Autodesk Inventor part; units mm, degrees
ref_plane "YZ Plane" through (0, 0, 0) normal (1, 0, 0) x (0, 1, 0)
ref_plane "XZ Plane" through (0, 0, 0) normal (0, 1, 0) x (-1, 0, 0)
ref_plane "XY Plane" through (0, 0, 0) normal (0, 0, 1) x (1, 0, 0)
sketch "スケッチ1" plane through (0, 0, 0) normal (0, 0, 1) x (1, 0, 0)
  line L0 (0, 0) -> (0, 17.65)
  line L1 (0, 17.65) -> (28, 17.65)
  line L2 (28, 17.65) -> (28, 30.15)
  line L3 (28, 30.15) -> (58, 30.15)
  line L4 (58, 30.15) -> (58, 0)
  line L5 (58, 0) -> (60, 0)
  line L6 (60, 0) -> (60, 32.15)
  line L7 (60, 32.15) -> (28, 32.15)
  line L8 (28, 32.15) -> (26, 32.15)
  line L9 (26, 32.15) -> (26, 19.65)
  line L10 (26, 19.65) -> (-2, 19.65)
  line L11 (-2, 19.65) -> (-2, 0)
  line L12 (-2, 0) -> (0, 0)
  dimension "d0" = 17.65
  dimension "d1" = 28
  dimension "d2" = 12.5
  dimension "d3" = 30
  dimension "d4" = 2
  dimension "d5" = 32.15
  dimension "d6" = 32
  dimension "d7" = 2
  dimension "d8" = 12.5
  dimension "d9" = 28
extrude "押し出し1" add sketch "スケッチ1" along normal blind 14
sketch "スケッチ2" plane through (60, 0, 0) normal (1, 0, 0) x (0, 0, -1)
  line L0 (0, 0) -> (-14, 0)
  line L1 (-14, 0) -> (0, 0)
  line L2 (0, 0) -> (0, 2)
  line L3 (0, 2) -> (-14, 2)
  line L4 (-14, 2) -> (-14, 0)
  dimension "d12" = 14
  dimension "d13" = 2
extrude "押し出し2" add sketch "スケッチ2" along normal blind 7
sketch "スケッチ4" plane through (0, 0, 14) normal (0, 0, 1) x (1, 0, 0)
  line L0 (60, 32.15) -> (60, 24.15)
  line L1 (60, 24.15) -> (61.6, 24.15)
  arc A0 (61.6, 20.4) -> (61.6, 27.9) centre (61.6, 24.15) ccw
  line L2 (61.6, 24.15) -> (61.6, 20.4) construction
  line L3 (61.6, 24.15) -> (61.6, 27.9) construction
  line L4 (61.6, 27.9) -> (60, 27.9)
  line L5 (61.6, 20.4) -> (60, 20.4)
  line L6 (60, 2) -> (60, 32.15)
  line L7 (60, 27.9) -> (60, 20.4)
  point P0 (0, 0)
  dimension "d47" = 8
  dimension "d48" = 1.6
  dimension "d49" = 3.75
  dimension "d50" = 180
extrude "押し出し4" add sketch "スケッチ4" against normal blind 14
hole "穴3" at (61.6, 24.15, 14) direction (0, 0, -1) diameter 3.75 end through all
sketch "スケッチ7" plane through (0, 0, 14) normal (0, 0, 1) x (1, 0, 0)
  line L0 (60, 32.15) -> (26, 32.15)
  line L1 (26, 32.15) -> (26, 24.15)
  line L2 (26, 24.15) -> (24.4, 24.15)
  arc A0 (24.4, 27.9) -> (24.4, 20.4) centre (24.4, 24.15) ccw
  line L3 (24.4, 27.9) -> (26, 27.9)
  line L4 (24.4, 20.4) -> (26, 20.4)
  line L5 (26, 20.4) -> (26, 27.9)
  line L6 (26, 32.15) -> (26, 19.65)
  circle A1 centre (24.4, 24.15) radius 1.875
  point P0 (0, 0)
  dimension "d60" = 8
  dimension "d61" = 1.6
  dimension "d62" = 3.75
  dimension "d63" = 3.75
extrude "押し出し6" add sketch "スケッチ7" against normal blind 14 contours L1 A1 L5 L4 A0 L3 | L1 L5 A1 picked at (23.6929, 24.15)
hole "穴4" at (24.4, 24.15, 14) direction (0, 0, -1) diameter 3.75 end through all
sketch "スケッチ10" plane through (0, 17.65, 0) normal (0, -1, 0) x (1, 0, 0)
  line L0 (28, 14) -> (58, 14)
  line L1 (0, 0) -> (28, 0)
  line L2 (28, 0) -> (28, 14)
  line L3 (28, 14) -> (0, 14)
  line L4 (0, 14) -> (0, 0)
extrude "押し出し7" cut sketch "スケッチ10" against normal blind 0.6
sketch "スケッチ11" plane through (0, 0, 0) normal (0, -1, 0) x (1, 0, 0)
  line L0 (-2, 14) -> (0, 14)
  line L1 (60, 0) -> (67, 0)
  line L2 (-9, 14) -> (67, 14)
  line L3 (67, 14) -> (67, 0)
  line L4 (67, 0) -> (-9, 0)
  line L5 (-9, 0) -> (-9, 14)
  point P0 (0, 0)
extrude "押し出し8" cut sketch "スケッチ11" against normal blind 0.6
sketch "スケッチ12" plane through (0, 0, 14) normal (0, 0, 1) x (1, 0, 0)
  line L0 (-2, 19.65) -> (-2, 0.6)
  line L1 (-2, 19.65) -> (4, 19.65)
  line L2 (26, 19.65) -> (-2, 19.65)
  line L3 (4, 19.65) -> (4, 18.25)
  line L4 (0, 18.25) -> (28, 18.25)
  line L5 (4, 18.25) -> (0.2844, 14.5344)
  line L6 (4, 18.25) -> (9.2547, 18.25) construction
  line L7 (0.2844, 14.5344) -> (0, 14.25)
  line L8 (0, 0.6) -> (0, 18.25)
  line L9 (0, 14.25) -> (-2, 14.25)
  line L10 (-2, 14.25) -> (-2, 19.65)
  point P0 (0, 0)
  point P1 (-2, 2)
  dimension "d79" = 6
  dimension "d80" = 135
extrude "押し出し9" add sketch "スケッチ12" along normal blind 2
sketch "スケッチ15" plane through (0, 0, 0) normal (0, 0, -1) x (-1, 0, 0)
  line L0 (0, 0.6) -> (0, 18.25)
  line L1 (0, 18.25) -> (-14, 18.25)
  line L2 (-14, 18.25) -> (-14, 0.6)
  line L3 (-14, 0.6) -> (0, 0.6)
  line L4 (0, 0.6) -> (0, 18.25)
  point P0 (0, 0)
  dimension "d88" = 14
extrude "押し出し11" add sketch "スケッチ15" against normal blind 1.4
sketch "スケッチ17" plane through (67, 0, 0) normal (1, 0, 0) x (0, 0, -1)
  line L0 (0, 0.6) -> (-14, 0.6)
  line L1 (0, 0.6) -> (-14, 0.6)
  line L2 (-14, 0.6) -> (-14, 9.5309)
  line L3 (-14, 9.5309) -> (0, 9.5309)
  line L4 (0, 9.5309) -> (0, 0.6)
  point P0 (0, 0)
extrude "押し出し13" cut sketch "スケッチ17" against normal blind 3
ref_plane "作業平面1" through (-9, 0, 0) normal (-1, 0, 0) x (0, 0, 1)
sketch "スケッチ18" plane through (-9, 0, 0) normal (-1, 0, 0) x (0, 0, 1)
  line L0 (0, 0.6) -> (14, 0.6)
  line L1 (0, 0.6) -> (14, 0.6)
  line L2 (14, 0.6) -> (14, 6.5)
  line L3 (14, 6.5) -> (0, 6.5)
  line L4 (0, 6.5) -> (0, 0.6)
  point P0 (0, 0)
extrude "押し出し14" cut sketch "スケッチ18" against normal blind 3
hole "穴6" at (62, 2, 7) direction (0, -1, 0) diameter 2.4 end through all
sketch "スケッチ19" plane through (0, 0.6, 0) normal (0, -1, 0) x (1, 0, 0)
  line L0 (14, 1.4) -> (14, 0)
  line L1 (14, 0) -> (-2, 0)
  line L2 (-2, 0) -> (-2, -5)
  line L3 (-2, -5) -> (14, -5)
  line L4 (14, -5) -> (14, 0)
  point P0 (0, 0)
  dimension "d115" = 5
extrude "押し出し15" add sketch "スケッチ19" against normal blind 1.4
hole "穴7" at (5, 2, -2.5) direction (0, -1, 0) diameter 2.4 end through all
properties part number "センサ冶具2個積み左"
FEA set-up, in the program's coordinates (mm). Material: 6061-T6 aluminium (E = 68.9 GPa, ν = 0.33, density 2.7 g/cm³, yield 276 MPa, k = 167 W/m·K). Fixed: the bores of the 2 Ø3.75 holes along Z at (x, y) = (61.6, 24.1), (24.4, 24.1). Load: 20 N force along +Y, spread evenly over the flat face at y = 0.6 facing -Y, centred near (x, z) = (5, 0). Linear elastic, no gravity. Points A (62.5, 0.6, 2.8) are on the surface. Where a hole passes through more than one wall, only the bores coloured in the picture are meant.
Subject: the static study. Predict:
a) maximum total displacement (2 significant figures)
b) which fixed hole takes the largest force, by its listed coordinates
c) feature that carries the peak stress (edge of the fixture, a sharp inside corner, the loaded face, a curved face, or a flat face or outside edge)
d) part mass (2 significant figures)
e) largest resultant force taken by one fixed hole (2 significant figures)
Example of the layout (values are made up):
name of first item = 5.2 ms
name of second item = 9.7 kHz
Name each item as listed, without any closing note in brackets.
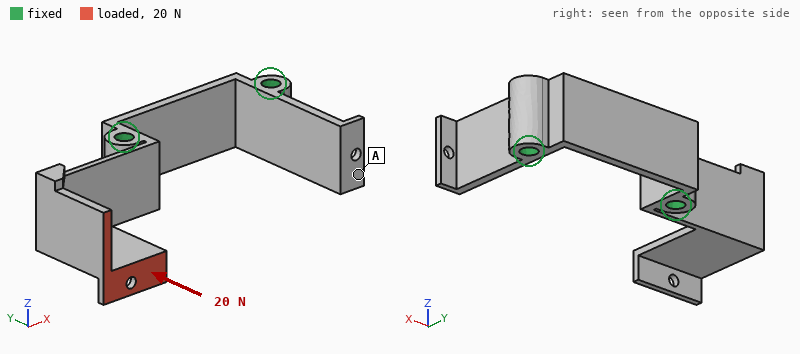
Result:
maximum total displacement = 0.70 mm
which fixed hole takes the largest force, by its listed coordinates = (24.4, 24.1)
feature that carries the peak stress = a flat face or outside edge
part mass = 12 g
largest resultant force taken by one fixed hole = 20 N
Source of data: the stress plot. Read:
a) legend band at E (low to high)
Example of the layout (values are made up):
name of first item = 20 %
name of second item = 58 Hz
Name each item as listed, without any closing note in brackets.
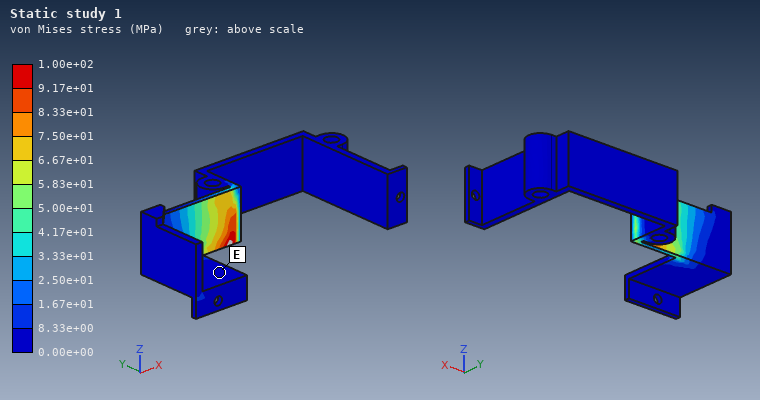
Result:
legend band at E = 0.00e+00 to 8.33e+00 MPa
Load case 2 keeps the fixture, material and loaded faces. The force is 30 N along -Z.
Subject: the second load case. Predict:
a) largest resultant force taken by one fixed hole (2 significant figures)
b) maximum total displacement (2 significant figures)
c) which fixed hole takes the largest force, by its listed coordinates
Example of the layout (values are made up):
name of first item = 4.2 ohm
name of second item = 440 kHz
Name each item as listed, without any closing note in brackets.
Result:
largest resultant force taken by one fixed hole = 30 N
maximum total displacement = 0.62 mm
which fixed hole takes the largest force, by its listed coordinates = (24.4, 24.1)
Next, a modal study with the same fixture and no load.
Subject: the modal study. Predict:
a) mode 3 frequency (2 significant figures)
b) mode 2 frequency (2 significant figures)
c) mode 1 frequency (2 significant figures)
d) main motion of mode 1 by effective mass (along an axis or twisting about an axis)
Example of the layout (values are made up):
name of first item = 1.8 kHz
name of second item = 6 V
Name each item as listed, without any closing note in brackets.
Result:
mode 3 frequency = 3200 Hz
mode 2 frequency = 1100 Hz
mode 1 frequency = 510 Hz
main motion of mode 1 by effective mass = along Y
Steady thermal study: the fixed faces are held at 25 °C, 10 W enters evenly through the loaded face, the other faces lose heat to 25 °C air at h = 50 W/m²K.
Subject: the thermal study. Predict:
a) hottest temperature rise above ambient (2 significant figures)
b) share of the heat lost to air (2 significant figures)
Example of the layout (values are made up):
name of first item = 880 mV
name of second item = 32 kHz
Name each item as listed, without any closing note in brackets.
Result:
hottest temperature rise above ambient = 68 K
share of the heat lost to air = 42 %
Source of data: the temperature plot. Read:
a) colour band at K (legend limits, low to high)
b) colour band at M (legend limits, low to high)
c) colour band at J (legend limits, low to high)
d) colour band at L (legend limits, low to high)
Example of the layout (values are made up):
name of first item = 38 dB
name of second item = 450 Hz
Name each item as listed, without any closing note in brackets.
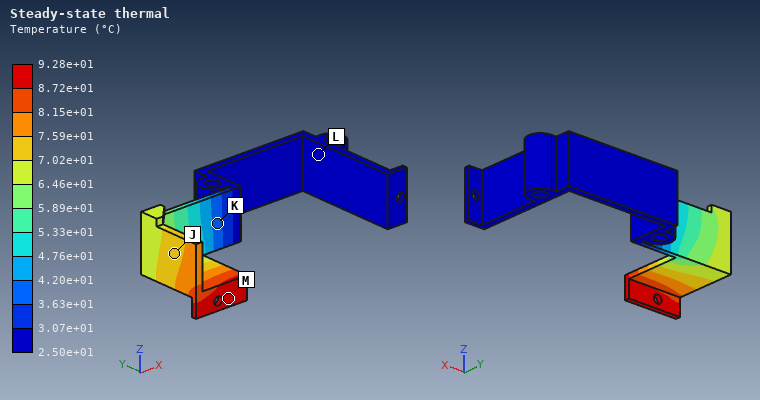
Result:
colour band at K = 3.63e+01 to 4.20e+01 °C
colour band at M = 8.72e+01 to 9.28e+01 °C
colour band at J = 7.02e+01 to 7.59e+01 °C
colour band at L = 2.50e+01 to 3.07e+01 °C
